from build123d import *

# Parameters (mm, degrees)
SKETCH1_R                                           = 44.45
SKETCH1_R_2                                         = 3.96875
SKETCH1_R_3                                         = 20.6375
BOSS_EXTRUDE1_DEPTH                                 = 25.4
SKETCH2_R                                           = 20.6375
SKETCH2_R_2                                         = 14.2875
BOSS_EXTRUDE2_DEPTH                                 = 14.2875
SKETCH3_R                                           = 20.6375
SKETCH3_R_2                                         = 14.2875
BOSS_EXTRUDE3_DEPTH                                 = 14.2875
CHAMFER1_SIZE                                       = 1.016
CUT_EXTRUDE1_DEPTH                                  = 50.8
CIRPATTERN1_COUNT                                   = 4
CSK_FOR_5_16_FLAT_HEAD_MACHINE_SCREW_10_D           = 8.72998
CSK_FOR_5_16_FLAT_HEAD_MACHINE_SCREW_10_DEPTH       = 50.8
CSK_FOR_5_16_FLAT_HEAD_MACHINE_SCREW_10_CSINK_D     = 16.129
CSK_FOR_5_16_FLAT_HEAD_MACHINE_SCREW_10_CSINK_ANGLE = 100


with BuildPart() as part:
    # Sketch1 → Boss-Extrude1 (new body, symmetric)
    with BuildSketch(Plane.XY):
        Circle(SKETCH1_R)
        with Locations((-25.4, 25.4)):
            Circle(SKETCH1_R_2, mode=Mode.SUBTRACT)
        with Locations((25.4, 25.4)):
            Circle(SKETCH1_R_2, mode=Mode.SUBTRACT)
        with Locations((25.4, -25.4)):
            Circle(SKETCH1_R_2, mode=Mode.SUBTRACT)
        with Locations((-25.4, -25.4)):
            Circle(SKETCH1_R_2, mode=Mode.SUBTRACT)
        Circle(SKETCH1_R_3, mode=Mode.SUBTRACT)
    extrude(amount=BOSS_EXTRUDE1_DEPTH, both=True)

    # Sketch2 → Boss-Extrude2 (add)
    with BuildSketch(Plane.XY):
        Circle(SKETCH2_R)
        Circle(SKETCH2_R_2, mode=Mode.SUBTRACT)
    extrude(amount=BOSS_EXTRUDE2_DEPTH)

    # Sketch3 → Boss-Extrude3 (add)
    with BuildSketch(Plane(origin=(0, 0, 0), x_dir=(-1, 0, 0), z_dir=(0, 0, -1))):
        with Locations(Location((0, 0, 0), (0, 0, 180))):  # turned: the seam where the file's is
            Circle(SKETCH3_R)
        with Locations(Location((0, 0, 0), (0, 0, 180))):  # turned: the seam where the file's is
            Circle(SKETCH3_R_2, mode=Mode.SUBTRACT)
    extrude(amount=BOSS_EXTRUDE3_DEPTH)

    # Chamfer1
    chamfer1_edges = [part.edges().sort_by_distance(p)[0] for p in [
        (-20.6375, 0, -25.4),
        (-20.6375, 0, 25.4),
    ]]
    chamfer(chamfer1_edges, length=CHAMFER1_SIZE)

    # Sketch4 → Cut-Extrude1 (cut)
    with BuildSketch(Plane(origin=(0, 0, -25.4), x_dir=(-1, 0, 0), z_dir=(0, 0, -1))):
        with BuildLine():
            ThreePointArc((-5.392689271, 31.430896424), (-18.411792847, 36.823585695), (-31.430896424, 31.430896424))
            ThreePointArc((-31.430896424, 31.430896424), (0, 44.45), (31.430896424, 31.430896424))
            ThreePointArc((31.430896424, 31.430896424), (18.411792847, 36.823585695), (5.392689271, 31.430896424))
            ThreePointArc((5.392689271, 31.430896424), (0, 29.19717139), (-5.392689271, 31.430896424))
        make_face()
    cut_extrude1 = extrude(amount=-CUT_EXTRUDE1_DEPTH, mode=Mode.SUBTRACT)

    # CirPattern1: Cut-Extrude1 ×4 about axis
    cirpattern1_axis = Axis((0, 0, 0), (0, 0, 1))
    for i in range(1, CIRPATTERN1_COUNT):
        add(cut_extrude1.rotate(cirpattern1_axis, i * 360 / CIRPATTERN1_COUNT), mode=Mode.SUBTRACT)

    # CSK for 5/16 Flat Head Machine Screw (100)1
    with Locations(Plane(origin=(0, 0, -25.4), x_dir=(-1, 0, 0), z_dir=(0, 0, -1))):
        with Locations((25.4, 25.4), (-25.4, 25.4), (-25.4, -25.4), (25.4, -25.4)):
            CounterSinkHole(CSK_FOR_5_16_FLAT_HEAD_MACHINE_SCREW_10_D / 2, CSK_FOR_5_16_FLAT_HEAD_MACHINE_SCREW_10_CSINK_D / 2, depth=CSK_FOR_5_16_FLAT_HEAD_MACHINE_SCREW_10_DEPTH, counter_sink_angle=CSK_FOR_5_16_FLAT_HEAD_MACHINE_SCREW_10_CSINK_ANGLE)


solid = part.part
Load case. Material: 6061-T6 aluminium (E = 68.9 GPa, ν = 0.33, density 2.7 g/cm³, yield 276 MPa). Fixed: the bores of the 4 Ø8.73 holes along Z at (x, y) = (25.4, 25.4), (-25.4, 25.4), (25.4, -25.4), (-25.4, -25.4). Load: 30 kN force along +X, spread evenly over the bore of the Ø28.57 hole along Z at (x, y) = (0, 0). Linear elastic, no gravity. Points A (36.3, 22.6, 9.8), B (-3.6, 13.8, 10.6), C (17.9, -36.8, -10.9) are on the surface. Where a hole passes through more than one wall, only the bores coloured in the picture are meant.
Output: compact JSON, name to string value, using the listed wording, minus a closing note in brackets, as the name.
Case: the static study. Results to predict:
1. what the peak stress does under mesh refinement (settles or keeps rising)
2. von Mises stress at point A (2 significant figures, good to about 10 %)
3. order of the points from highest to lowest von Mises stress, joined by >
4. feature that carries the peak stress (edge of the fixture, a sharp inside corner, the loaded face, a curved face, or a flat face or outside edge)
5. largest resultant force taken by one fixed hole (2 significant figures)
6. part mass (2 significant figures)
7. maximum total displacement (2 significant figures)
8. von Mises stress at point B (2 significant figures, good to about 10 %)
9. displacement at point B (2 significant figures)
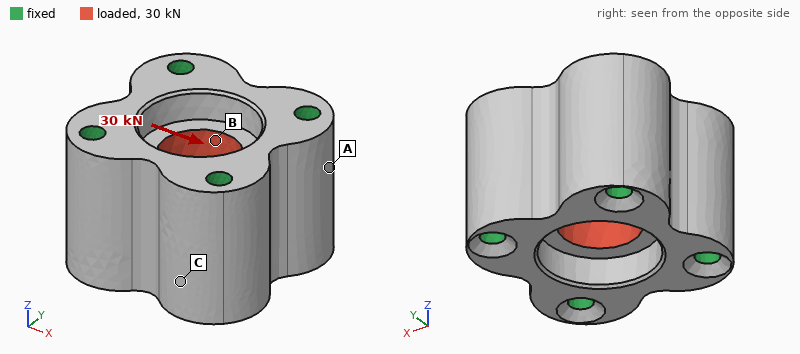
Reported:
{"what the peak stress does under mesh refinement": "keeps rising", "von Mises stress at point A": "5.2 MPa", "order of the points from highest to lowest von Mises stress, joined by >": "B > A > C", "feature that carries the peak stress": "edge of the fixture", "largest resultant force taken by one fixed hole": "8.3 kN", "part mass": "470 g", "maximum total displacement": "6.5 µm", "von Mises stress at point B": "21 MPa", "displacement at point B": "3.9 µm"}
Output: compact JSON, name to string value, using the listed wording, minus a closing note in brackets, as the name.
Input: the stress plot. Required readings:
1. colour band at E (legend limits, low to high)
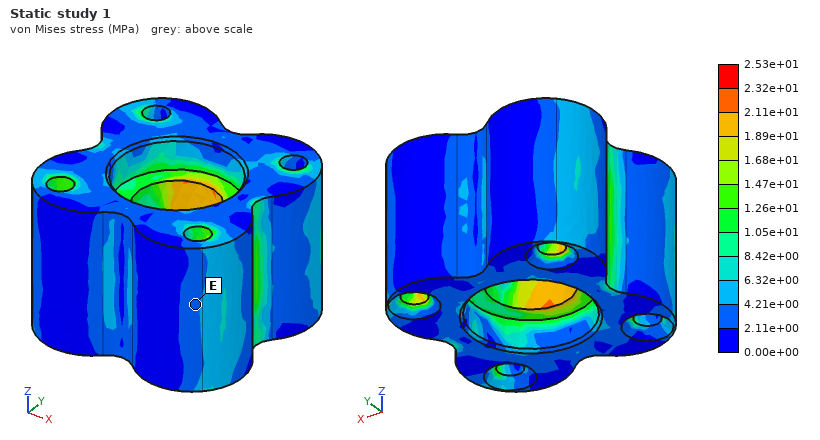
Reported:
{"colour band at E": "2.11e+00 to 4.21e+00 MPa"}
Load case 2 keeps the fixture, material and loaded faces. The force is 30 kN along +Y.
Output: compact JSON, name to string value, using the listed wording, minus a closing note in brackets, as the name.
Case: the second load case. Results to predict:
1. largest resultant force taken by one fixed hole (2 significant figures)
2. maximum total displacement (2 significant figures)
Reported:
{"largest resultant force taken by one fixed hole": "8.3 kN", "maximum total displacement": "6.4 µm"}
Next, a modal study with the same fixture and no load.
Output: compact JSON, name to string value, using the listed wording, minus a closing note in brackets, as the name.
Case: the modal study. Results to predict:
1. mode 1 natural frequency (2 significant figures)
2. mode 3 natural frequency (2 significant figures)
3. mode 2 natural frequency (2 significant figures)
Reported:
{"mode 1 natural frequency": "22 kHz", "mode 3 natural frequency": "29 kHz", "mode 2 natural frequency": "29 kHz"}
